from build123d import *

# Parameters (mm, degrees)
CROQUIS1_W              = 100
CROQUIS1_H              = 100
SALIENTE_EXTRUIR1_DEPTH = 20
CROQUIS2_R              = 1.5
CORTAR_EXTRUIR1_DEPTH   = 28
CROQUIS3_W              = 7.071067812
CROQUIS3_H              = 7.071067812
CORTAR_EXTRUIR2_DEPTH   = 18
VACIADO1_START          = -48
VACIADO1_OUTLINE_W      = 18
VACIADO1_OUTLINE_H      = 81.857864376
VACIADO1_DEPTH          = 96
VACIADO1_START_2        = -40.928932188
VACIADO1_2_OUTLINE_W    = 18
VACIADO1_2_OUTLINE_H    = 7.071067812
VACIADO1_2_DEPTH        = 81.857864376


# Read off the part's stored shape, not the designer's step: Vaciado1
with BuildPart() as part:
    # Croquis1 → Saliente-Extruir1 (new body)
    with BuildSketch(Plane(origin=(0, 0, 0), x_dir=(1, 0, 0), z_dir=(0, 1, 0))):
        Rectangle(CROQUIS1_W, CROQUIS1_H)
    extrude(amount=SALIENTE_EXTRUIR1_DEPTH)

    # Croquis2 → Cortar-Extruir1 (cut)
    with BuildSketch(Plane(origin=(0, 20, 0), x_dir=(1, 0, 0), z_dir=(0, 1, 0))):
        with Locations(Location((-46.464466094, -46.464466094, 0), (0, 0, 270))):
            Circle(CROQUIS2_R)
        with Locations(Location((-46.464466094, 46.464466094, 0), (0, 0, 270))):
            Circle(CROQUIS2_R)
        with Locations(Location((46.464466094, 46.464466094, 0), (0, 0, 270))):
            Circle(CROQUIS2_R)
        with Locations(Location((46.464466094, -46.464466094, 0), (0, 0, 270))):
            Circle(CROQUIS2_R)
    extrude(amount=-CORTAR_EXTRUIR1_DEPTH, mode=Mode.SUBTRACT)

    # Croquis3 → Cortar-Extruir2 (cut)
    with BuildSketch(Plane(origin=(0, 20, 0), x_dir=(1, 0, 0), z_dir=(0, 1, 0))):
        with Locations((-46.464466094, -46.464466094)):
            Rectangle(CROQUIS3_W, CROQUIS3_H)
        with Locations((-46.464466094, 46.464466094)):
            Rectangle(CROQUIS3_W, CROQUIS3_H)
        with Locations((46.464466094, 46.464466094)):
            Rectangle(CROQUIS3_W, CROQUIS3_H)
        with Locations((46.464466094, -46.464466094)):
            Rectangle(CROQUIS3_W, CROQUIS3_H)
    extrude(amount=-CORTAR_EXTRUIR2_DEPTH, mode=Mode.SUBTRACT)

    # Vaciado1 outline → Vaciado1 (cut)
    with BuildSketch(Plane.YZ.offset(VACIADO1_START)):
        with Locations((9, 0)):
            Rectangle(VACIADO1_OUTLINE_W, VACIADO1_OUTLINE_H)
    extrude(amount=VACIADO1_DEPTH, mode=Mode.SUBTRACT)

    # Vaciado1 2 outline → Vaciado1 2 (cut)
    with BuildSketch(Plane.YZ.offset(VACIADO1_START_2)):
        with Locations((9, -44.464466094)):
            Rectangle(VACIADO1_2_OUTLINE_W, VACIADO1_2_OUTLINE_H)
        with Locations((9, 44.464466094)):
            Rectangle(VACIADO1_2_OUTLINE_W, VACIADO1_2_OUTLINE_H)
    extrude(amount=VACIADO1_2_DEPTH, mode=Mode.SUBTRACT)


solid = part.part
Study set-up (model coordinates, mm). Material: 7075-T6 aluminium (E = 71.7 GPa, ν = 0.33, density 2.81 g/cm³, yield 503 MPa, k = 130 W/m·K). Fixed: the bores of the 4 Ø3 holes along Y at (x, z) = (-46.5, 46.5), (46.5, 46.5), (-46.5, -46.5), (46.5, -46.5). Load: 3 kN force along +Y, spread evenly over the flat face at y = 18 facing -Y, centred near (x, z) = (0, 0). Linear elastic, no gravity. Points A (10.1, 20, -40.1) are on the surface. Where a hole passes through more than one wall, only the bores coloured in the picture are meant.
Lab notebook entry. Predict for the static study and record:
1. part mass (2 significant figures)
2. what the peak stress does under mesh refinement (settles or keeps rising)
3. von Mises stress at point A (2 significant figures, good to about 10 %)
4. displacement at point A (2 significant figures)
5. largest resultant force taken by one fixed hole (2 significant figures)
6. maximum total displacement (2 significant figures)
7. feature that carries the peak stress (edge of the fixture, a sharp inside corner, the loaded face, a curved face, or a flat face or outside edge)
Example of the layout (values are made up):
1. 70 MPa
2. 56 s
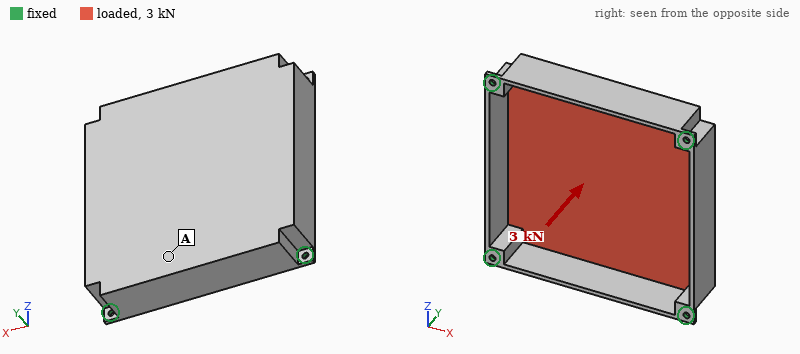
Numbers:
1. 96 g
2. keeps rising
3. 57 MPa
4. 0.33 mm
5. 970 N
6. 1.3 mm
7. edge of the fixture
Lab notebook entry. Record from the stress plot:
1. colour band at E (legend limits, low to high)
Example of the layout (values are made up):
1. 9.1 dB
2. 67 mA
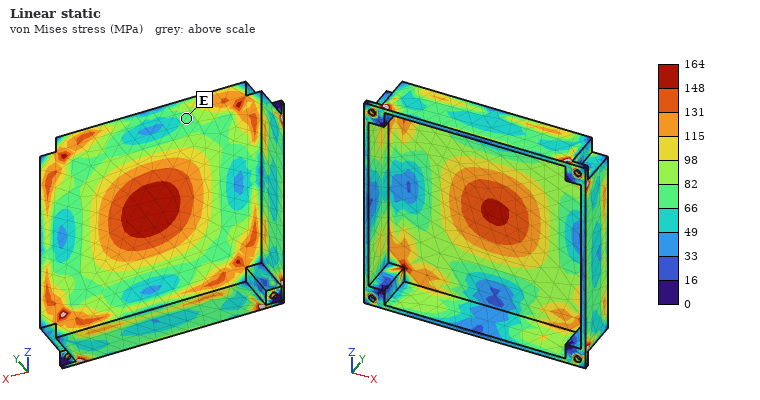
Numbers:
1. 66 to 82 MPa
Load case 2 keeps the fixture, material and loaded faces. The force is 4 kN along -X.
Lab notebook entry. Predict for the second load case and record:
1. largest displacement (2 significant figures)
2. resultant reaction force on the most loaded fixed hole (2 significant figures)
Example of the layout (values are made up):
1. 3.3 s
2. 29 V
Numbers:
1. 48 µm
2. 1.1 kN
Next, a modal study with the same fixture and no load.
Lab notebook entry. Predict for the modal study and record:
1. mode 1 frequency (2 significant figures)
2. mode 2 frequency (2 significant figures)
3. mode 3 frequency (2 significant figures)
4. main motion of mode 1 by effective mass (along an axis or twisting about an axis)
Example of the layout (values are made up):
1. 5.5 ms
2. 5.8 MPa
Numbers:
1. 1300 Hz
2. 2700 Hz
3. 2700 Hz
4. along Y
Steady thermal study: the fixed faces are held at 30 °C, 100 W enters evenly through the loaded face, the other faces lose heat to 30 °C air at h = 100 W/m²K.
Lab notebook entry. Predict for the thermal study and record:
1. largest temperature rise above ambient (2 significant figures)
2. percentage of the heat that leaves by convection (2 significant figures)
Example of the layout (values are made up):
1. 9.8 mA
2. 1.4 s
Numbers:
1. 47 K
2. 71 %
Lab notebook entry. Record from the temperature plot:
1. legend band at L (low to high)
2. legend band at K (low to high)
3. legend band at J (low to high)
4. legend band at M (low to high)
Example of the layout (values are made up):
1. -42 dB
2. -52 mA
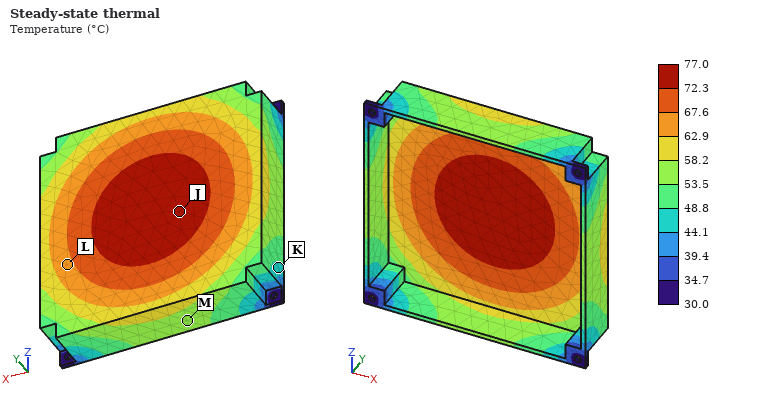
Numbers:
1. 62.9 to 67.6 °C
2. 44.1 to 48.8 °C
3. 72.3 to 77.0 °C
4. 53.5 to 58.2 °C
